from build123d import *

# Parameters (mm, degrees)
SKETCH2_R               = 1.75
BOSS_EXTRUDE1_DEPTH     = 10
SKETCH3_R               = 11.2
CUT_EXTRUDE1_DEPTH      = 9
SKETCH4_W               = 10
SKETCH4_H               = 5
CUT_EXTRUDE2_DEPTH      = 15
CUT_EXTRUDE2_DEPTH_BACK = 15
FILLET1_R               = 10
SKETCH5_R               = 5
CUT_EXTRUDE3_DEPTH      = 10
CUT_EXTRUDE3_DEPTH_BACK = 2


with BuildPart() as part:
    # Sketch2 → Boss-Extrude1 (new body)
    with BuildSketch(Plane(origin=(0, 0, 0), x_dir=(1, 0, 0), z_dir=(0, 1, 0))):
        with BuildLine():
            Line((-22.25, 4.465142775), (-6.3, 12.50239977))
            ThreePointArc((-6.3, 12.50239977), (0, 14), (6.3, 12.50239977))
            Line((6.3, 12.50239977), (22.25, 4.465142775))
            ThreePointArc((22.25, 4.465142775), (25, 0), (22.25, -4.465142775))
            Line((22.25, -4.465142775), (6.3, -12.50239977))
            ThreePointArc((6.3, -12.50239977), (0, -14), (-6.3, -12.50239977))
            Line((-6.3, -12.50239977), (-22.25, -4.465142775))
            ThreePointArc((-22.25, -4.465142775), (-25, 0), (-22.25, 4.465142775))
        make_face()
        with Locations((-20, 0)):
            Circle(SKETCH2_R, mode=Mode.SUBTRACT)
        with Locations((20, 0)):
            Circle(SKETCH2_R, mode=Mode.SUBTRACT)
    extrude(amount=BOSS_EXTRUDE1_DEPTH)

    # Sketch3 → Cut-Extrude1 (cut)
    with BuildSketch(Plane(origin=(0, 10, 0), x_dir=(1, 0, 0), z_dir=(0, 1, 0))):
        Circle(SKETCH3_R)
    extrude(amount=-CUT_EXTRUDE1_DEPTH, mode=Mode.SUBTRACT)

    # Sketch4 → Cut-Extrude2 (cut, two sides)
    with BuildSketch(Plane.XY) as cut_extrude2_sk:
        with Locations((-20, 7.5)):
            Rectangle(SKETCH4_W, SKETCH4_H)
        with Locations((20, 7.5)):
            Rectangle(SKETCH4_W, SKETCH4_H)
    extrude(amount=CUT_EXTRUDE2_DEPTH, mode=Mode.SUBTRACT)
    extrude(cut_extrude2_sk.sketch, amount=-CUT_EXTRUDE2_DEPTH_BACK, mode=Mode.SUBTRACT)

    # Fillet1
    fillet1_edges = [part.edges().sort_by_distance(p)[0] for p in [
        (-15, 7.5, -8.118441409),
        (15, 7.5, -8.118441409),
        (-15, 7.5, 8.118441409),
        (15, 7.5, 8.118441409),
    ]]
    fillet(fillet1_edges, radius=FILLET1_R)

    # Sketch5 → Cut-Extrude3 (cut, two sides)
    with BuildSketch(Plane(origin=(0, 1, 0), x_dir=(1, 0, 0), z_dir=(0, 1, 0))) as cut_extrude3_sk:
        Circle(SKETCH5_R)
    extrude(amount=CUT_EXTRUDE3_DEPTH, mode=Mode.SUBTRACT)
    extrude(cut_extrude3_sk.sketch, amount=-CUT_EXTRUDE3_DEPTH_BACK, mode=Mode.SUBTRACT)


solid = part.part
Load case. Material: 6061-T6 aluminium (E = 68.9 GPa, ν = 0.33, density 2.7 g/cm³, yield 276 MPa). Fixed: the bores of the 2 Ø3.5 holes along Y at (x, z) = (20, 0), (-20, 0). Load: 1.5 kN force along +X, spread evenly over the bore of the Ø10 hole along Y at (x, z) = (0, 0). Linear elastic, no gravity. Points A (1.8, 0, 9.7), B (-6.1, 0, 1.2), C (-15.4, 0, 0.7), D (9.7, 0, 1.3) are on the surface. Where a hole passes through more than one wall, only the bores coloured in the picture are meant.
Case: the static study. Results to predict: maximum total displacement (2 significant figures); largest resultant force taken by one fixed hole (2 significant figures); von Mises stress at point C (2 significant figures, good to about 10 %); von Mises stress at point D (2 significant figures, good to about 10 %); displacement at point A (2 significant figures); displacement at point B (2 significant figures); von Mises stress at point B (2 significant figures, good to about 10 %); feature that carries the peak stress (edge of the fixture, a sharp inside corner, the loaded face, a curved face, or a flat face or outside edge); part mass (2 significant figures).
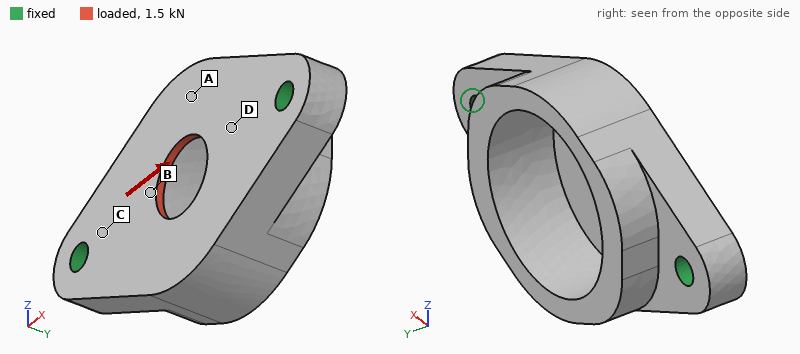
9.4 µm
750 N
25 MPa
48 MPa
4.0 µm
7.5 µm
53 MPa
the loaded face
11 g
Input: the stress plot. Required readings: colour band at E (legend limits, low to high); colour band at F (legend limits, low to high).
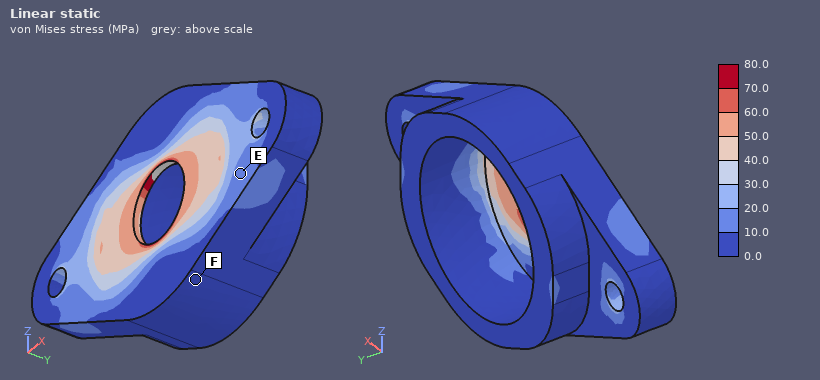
10.0 to 20.0 MPa
0.0 to 10.0 MPa
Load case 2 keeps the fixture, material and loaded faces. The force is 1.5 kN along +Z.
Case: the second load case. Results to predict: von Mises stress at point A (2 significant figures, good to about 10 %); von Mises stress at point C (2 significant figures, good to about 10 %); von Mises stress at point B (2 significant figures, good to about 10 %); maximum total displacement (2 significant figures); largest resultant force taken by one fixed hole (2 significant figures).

42 MPa
31 MPa
51 MPa
21 µm
750 N
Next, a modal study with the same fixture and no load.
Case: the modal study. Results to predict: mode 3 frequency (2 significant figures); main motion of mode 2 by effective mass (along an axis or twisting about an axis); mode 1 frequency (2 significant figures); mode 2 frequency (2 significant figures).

22 kHz
along Y
11 kHz
13 kHz
